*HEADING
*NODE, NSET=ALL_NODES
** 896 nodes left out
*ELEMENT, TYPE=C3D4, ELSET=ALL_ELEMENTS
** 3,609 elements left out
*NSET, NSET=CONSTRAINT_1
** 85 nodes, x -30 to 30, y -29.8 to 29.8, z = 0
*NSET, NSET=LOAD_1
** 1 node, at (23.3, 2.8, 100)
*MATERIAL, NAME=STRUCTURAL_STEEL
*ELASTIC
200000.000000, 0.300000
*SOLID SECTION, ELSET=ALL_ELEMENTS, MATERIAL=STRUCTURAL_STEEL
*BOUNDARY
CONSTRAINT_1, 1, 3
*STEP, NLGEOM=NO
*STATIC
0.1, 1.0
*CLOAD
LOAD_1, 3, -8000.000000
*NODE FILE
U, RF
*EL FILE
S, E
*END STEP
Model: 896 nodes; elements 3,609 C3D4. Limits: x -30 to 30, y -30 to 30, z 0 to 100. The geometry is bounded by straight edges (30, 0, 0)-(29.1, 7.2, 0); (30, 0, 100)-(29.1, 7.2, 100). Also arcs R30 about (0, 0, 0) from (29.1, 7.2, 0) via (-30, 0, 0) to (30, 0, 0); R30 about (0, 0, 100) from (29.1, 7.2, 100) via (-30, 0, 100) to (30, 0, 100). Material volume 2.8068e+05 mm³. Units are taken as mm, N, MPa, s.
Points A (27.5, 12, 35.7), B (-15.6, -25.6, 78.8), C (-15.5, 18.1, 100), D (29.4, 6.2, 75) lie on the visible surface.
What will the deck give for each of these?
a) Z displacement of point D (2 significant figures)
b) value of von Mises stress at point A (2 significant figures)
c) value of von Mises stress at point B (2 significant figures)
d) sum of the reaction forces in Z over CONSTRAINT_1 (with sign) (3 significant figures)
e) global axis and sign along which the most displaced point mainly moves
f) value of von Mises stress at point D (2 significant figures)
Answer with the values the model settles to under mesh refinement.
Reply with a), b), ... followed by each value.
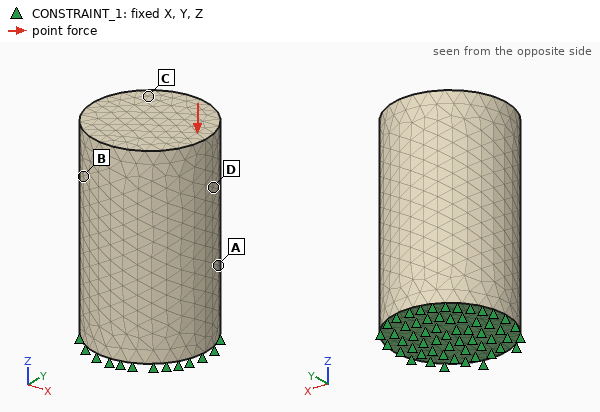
a) -0.0048 mm
b) 11 MPa
c) 2.8 MPa
d) 8000 N
e) -Z
f) 20 MPa
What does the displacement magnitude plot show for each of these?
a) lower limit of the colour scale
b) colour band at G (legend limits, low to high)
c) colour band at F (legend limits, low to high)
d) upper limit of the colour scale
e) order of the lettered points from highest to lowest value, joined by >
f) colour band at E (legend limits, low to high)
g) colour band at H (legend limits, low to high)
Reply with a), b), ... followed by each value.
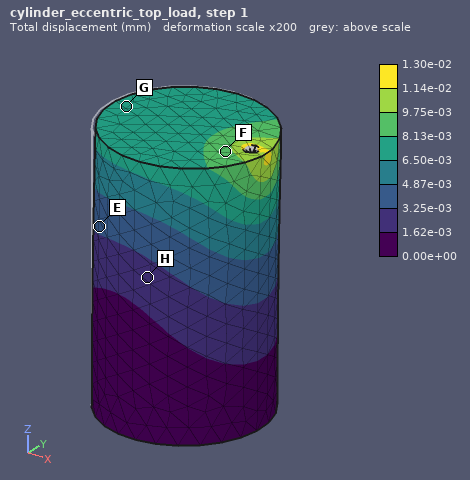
a) 0.00e+00 mm
b) 6.50e-03 to 8.13e-03 mm
c) 8.13e-03 to 9.75e-03 mm
d) 1.30e-02 mm
e) F > G > E > H
f) 3.25e-03 to 4.87e-03 mm
g) 1.62e-03 to 3.25e-03 mm
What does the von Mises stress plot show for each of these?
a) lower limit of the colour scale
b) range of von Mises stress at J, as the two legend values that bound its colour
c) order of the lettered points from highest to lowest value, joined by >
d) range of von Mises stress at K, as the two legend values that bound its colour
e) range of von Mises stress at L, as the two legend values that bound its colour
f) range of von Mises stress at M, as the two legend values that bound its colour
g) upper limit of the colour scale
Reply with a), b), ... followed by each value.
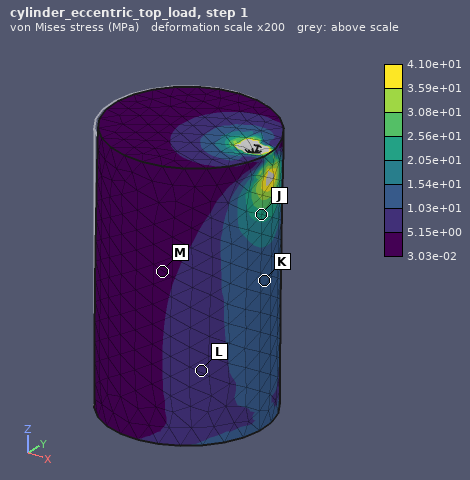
a) 3.03e-02 MPa
b) 2.05e+01 to 2.56e+01 MPa
c) J > K > L > M
d) 1.03e+01 to 1.54e+01 MPa
e) 5.15e+00 to 1.03e+01 MPa
f) 3.03e-02 to 5.15e+00 MPa
g) 4.10e+01 MPa
